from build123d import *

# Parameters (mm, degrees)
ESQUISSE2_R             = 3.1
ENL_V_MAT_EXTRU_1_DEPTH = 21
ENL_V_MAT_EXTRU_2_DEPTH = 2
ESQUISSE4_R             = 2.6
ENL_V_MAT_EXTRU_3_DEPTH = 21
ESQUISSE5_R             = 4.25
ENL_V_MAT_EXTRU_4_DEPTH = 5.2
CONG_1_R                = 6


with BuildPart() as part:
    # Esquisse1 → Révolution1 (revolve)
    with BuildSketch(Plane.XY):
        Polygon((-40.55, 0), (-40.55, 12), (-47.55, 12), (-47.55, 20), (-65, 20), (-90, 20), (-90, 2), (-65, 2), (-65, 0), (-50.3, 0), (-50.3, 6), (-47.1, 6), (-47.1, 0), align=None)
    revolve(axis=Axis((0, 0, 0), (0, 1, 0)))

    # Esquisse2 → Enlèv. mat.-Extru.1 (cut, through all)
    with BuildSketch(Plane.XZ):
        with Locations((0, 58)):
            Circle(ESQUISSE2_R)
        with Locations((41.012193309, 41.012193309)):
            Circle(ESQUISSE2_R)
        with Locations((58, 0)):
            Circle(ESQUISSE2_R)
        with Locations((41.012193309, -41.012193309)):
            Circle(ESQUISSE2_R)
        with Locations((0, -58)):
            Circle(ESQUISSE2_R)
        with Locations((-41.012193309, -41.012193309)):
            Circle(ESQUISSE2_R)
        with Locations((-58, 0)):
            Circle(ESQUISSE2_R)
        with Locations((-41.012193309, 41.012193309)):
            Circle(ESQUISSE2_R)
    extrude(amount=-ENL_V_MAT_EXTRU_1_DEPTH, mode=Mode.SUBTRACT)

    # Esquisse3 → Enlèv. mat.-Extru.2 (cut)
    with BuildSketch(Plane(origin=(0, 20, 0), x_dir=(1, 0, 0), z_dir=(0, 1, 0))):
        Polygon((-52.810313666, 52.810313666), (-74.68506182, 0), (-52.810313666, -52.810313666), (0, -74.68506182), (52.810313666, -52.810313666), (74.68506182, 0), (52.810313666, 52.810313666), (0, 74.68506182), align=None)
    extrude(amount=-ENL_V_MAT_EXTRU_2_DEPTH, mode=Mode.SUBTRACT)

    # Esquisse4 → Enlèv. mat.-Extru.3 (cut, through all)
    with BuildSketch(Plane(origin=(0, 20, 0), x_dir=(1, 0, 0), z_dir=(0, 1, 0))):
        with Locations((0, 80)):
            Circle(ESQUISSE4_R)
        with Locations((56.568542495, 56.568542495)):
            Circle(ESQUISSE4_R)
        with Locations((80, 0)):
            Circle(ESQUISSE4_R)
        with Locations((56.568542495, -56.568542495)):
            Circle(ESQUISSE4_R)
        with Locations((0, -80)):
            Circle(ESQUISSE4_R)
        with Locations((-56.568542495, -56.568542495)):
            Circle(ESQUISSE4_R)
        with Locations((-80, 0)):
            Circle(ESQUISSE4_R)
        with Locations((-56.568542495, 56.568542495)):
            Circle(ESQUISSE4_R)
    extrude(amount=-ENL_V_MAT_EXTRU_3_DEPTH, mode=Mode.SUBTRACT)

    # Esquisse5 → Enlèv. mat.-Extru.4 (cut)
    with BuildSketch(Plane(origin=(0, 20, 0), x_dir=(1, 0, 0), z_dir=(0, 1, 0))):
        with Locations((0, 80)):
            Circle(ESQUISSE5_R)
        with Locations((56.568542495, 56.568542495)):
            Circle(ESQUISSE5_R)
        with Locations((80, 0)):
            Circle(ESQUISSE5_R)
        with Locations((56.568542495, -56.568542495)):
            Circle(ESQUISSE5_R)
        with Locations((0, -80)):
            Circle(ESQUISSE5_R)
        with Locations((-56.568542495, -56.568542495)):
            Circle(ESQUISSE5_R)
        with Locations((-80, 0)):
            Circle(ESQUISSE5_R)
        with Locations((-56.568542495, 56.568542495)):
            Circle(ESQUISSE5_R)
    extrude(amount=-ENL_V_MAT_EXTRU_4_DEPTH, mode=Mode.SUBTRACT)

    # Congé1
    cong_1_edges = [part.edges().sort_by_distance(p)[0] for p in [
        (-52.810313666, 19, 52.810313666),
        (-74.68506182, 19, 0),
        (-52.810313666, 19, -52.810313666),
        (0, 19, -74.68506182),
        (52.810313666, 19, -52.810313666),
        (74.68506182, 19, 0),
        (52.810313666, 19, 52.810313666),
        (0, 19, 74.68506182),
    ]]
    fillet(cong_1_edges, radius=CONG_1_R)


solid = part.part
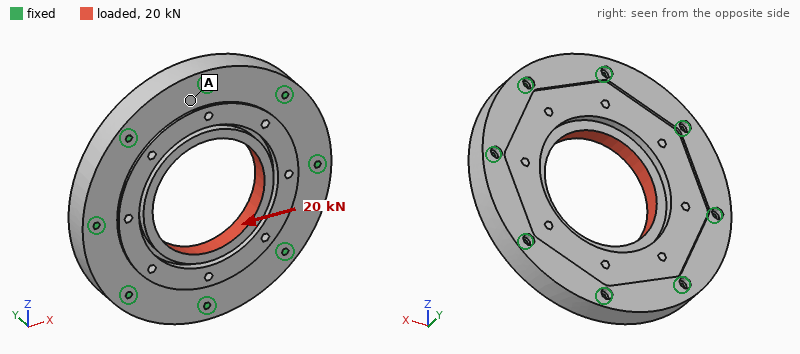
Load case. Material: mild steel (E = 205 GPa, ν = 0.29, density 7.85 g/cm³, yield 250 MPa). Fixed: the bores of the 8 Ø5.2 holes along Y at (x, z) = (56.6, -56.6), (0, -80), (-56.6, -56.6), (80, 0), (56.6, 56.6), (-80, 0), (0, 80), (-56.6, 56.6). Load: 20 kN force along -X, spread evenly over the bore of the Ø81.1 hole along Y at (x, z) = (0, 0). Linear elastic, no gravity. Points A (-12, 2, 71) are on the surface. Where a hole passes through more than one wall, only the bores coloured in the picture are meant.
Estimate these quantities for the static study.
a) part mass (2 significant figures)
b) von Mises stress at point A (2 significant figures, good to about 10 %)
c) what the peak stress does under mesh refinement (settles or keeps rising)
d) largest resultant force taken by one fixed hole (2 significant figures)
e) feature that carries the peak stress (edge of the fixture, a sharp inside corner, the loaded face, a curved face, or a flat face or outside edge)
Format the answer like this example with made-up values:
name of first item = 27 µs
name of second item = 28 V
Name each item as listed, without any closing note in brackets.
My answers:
part mass = 2.6 kg
von Mises stress at point A = 2.9 MPa
what the peak stress does under mesh refinement = keeps rising
largest resultant force taken by one fixed hole = 3.4 kN
feature that carries the peak stress = edge of the fixture
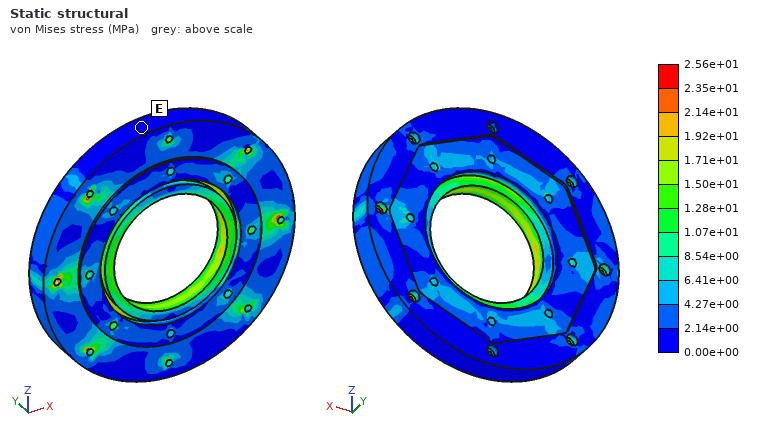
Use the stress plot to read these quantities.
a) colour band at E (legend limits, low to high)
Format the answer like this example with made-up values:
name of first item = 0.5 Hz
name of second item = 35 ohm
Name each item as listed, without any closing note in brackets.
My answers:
colour band at E = 0.00e+00 to 2.14e+00 MPa
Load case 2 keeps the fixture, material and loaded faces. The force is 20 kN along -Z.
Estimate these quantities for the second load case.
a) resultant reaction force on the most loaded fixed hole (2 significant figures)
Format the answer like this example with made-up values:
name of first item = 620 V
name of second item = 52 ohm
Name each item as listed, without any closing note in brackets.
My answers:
resultant reaction force on the most loaded fixed hole = 3.4 kN
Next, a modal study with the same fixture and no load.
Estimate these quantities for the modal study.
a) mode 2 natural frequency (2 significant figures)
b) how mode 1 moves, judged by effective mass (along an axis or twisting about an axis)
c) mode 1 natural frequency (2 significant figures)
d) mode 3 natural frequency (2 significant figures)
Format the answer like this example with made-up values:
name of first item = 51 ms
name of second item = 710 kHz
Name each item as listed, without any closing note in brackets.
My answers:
mode 2 natural frequency = 7900 Hz
how mode 1 moves, judged by effective mass = along Y
mode 1 natural frequency = 6200 Hz
mode 3 natural frequency = 7900 Hz
